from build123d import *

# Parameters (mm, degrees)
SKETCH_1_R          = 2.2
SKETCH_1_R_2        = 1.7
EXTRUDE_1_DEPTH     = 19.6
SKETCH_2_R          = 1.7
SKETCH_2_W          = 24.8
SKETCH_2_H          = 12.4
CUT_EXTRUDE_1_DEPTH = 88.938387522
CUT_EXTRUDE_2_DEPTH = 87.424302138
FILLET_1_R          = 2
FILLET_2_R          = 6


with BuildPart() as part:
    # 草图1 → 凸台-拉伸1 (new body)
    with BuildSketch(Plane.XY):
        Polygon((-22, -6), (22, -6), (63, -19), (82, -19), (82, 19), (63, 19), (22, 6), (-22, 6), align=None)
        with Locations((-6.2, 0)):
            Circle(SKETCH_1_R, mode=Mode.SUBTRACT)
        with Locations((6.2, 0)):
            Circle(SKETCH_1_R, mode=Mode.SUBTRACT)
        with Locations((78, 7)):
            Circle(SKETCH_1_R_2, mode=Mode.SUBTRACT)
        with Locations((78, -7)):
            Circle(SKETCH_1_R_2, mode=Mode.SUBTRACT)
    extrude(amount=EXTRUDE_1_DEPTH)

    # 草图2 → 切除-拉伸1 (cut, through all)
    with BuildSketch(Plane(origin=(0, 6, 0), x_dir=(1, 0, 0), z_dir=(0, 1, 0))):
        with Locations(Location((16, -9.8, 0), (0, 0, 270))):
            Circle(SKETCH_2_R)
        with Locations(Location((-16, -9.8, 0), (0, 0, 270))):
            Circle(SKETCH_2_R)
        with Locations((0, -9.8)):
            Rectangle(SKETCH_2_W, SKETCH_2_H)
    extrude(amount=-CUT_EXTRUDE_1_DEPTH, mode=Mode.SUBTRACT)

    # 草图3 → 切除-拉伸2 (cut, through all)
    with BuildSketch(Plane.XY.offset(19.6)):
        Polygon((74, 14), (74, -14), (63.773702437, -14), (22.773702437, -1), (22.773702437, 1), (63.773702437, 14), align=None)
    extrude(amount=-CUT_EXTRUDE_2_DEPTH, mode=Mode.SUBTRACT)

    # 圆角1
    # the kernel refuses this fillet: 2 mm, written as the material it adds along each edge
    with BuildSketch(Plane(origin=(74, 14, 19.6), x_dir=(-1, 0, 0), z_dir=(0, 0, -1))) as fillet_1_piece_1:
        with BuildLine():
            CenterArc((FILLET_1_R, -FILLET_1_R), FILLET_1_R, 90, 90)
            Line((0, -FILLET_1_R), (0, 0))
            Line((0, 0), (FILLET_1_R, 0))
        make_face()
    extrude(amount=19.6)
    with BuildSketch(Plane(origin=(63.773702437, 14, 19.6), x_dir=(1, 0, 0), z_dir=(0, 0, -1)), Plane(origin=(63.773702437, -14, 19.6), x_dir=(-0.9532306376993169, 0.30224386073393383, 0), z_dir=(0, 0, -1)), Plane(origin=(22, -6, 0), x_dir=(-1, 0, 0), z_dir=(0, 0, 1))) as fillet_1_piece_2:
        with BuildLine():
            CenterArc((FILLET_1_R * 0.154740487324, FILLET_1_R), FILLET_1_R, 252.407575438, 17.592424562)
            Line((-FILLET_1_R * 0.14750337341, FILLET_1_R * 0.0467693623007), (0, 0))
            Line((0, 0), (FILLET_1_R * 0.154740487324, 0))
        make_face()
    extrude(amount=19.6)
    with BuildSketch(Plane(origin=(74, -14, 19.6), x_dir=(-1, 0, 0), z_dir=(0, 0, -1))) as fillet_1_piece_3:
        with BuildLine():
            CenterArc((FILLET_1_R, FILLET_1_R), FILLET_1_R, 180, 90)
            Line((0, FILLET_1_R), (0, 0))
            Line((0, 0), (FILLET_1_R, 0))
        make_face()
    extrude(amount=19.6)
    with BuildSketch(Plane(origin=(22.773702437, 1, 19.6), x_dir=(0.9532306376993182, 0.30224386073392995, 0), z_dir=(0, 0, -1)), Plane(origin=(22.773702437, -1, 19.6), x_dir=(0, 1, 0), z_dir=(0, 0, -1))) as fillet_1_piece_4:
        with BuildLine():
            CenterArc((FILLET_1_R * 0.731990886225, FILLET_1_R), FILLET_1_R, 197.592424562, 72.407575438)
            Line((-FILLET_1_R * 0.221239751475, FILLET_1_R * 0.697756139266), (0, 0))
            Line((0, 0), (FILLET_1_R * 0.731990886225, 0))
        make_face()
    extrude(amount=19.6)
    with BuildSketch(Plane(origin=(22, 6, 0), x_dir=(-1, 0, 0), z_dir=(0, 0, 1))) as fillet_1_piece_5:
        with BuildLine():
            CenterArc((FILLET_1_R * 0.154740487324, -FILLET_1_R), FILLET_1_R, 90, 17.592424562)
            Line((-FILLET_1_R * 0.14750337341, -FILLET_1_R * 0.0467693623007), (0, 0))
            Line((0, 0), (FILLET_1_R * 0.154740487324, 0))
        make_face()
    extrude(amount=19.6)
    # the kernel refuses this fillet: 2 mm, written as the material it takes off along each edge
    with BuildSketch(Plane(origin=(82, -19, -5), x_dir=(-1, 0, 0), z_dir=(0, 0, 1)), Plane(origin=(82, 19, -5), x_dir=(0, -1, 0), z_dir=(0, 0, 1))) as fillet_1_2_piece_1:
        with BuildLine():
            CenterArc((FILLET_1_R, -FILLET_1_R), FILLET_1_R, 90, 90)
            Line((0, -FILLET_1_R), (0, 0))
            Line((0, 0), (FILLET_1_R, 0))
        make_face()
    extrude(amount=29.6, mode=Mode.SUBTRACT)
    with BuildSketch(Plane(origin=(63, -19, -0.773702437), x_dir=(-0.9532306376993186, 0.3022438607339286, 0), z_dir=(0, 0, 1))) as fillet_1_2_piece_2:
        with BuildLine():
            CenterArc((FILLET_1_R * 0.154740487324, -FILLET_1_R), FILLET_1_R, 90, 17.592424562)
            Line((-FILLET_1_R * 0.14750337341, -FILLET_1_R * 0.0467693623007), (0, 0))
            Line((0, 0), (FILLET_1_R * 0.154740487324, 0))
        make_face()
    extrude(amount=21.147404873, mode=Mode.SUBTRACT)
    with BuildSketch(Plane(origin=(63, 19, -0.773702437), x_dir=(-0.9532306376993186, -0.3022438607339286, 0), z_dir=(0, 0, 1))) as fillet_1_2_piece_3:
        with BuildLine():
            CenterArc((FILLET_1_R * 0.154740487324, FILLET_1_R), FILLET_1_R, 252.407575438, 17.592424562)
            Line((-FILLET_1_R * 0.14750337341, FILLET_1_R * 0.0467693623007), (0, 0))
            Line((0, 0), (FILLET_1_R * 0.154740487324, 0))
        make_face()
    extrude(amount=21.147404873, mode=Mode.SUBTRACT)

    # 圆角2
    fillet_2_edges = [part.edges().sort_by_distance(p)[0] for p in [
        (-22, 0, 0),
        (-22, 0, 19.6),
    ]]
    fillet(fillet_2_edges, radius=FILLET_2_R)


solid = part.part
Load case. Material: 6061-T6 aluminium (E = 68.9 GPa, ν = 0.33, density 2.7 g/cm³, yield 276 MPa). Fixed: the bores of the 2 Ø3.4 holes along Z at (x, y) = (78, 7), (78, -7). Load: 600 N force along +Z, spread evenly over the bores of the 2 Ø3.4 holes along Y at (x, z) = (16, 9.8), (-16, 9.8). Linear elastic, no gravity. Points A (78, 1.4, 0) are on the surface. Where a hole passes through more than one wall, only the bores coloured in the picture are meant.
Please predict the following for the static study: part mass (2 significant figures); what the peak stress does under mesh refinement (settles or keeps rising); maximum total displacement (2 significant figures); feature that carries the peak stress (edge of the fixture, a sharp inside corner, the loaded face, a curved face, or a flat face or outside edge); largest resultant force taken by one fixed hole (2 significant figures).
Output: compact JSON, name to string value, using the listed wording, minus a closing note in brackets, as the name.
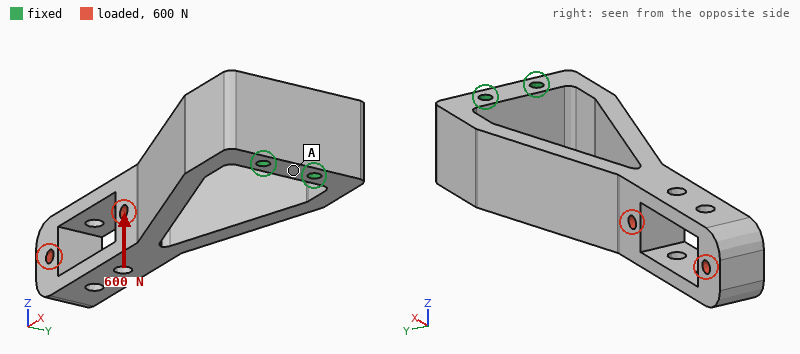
{"part mass": "60 g", "what the peak stress does under mesh refinement": "keeps rising", "maximum total displacement": "0.72 mm", "feature that carries the peak stress": "edge of the fixture", "largest resultant force taken by one fixed hole": "300 N"}
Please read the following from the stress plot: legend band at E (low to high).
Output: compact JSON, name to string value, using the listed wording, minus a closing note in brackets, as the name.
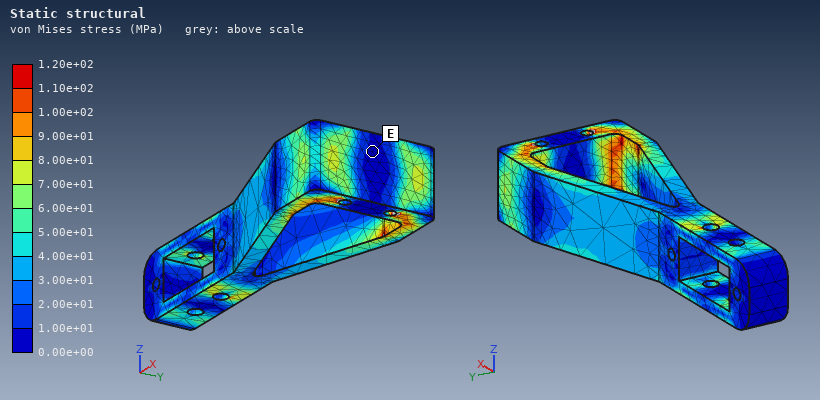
{"legend band at E": "0.00e+00 to 1.00e+01 MPa"}
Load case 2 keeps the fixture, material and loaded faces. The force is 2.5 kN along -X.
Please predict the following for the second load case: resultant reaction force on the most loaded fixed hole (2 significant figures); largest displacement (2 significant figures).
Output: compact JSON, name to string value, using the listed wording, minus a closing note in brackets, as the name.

{"resultant reaction force on the most loaded fixed hole": "1.3 kN", "largest displacement": "44 µm"}
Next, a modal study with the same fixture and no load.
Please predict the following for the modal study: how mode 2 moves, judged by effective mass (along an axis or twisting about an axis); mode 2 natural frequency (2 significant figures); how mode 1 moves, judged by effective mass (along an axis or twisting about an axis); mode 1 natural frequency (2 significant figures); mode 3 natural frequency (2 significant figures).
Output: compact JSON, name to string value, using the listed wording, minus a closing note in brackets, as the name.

{"how mode 2 moves, judged by effective mass": "along Y", "mode 2 natural frequency": "2100 Hz", "how mode 1 moves, judged by effective mass": "along Z", "mode 1 natural frequency": "1200 Hz", "mode 3 natural frequency": "2800 Hz"}
